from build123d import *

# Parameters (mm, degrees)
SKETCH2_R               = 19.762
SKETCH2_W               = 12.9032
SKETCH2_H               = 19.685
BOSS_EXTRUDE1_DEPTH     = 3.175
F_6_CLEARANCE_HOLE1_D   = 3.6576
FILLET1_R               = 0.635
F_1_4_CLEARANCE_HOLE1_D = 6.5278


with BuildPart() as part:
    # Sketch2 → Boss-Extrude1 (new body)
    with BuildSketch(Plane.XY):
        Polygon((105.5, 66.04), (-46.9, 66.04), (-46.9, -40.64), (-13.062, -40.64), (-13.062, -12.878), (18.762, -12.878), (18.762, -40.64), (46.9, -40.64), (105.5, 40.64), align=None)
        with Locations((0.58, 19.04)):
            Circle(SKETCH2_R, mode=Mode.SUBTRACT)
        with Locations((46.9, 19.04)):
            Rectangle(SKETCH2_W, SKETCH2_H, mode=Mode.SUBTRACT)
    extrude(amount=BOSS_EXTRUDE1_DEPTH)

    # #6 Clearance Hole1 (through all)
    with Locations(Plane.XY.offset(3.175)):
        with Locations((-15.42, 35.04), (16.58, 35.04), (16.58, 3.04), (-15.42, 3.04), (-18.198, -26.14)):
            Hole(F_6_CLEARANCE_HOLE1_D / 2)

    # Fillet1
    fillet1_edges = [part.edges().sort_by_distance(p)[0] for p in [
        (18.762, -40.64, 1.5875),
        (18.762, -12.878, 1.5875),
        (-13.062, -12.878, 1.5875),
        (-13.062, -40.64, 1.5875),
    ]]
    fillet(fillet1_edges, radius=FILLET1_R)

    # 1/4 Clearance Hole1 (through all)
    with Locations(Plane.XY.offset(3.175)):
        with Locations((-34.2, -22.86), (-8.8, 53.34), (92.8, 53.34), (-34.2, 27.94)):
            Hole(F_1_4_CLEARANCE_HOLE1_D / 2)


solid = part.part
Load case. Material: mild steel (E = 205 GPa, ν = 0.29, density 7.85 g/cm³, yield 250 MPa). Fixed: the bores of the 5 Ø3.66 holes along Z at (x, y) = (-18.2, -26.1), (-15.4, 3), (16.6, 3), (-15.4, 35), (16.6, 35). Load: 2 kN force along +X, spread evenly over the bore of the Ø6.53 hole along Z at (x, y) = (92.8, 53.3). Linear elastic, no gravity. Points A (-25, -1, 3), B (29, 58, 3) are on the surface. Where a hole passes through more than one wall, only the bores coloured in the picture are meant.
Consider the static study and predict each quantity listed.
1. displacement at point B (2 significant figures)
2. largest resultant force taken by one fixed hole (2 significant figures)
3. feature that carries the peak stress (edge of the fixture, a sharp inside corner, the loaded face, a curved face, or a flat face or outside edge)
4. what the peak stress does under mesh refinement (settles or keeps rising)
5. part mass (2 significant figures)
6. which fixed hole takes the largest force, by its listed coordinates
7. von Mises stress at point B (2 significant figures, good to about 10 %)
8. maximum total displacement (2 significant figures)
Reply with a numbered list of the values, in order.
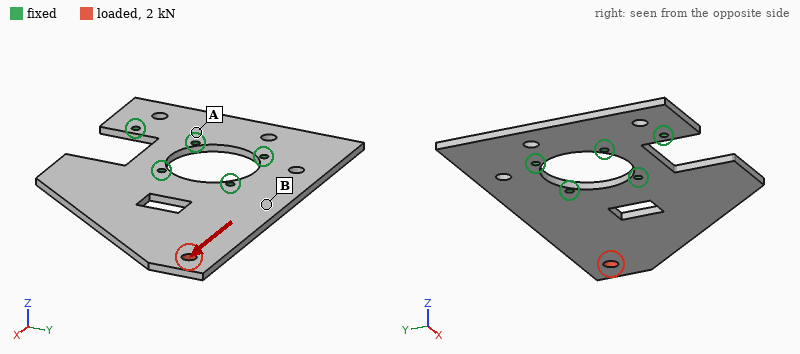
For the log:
1. 5.4 µm
2. 1.7 kN
3. edge of the fixture
4. keeps rising
5. 280 g
6. (16.6, 35)
7. 18 MPa
8. 20 µm
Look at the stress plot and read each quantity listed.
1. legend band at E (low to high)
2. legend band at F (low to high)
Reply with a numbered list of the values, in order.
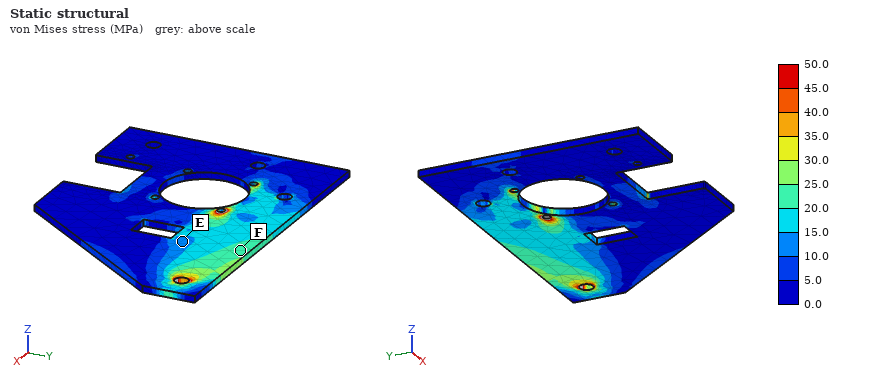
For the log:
1. 10.0 to 15.0 MPa
2. 20.0 to 25.0 MPa
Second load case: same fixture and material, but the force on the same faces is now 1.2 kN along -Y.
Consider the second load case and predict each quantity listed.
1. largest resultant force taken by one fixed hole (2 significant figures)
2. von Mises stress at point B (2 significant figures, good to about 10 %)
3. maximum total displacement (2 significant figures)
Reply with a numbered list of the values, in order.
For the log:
1. 1.5 kN
2. 17 MPa
3. 30 µm
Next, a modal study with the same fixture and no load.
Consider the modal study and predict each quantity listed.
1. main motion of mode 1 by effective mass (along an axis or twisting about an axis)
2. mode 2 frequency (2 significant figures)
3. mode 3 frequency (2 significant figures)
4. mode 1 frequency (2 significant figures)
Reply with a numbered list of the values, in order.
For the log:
1. along Z
2. 890 Hz
3. 1500 Hz
4. 380 Hz
